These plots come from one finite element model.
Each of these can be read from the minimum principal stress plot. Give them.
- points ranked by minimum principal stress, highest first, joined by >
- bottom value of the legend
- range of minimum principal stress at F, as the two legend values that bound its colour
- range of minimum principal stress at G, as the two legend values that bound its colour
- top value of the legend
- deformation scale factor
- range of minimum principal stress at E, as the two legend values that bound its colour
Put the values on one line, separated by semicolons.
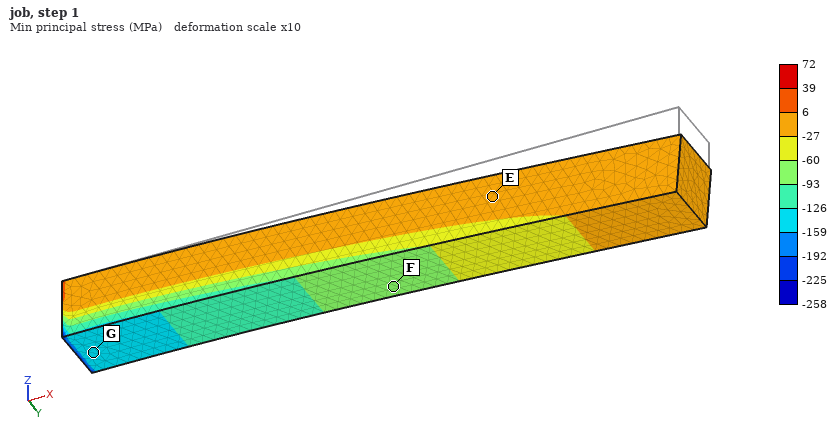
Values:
E > F > G; -258 MPa; -93 to -60 MPa; -159 to -126 MPa; 72 MPa; 10; -27 to 6 MPa
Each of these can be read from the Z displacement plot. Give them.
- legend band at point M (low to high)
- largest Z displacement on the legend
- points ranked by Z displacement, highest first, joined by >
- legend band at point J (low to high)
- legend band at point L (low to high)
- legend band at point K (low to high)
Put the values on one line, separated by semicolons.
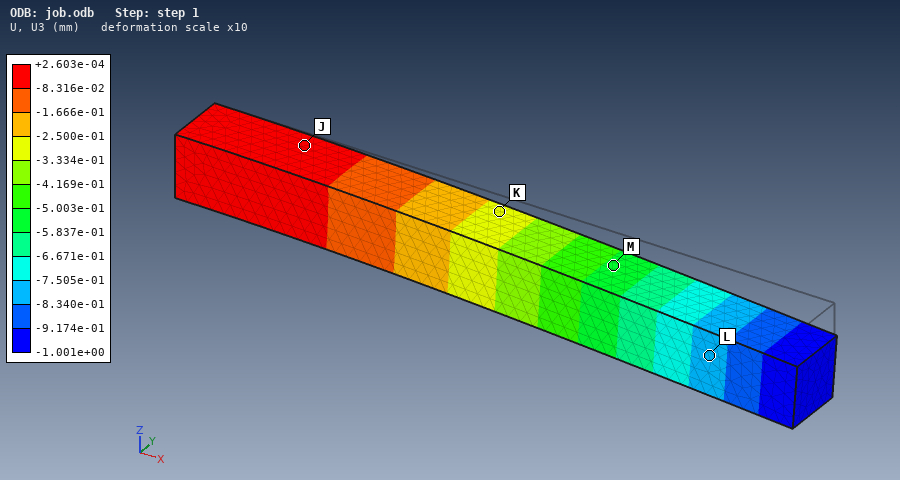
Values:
-5.837e-01 to -5.003e-01 mm; +2.603e-04 mm; J > K > M > L; -8.316e-02 to +2.603e-04 mm; -8.340e-01 to -7.505e-01 mm; -3.334e-01 to -2.500e-01 mm
